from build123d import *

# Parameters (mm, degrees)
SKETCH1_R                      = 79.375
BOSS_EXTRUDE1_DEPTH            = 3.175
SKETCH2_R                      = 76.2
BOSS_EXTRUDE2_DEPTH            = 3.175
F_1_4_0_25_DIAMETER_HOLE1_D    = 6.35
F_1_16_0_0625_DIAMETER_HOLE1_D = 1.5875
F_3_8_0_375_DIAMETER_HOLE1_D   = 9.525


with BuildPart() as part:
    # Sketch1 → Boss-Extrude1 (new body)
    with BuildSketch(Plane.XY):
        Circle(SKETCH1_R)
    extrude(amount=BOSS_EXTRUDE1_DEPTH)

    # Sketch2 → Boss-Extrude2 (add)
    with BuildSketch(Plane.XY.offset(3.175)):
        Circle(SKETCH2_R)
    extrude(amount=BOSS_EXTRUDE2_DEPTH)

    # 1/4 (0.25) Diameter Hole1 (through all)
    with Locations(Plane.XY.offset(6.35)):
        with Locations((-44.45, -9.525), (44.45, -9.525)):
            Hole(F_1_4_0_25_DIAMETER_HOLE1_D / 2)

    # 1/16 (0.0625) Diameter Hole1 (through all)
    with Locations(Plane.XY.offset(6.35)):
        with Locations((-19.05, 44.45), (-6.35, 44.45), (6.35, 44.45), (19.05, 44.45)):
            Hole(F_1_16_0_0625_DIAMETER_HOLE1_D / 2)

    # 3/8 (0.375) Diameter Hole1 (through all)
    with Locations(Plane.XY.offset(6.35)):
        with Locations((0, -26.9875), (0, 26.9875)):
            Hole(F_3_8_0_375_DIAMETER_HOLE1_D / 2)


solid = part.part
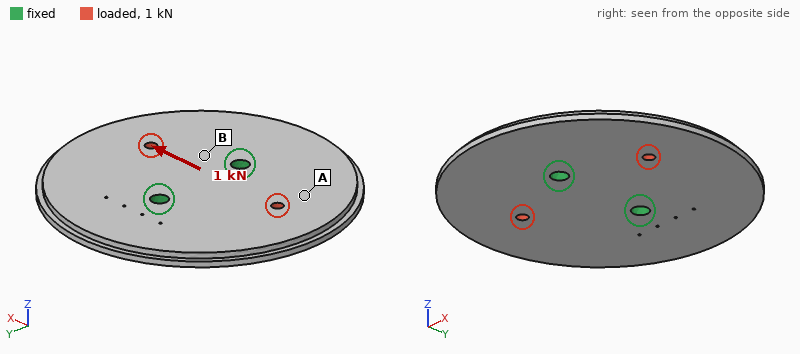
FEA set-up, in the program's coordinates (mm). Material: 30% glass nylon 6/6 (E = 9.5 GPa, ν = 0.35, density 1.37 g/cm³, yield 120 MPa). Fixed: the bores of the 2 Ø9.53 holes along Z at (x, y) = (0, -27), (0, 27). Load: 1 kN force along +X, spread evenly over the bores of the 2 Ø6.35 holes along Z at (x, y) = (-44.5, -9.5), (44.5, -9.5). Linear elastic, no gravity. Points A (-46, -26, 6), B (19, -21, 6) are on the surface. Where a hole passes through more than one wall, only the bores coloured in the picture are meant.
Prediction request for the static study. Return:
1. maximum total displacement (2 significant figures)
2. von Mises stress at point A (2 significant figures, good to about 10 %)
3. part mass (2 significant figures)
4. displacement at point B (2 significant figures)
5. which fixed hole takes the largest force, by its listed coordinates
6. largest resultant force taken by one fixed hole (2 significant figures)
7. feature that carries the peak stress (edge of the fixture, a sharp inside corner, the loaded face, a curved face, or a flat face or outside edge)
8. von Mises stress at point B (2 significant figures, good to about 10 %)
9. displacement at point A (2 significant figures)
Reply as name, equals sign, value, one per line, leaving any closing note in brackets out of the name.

maximum total displacement = 12 µm
von Mises stress at point A = 0.84 MPa
part mass = 160 g
displacement at point B = 4.2 µm
which fixed hole takes the largest force, by its listed coordinates = (0, -27)
largest resultant force taken by one fixed hole = 670 N
feature that carries the peak stress = the loaded face
von Mises stress at point B = 2.1 MPa
displacement at point A = 7.3 µm
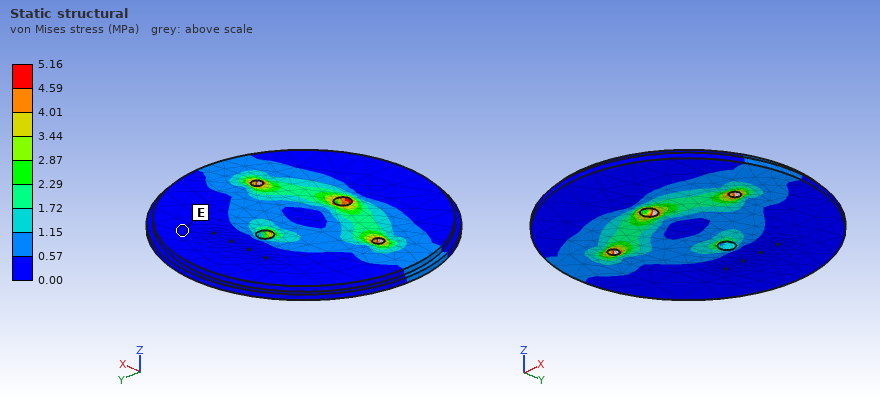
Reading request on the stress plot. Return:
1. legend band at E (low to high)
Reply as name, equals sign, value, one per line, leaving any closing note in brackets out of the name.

legend band at E = 0.00 to 0.57 MPa
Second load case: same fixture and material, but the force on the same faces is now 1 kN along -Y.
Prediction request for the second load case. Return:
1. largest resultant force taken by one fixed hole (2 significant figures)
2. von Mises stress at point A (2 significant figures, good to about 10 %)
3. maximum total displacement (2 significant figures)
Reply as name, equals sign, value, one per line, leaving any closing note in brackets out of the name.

largest resultant force taken by one fixed hole = 520 N
von Mises stress at point A = 1.3 MPa
maximum total displacement = 14 µm
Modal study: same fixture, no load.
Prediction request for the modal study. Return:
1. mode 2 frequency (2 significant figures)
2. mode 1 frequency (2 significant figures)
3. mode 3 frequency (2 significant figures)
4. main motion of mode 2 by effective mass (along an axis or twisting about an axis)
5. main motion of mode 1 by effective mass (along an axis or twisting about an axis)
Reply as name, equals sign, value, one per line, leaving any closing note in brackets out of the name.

mode 2 frequency = 620 Hz
mode 1 frequency = 510 Hz
mode 3 frequency = 890 Hz
main motion of mode 2 by effective mass = along Z
main motion of mode 1 by effective mass = twisting about Y
